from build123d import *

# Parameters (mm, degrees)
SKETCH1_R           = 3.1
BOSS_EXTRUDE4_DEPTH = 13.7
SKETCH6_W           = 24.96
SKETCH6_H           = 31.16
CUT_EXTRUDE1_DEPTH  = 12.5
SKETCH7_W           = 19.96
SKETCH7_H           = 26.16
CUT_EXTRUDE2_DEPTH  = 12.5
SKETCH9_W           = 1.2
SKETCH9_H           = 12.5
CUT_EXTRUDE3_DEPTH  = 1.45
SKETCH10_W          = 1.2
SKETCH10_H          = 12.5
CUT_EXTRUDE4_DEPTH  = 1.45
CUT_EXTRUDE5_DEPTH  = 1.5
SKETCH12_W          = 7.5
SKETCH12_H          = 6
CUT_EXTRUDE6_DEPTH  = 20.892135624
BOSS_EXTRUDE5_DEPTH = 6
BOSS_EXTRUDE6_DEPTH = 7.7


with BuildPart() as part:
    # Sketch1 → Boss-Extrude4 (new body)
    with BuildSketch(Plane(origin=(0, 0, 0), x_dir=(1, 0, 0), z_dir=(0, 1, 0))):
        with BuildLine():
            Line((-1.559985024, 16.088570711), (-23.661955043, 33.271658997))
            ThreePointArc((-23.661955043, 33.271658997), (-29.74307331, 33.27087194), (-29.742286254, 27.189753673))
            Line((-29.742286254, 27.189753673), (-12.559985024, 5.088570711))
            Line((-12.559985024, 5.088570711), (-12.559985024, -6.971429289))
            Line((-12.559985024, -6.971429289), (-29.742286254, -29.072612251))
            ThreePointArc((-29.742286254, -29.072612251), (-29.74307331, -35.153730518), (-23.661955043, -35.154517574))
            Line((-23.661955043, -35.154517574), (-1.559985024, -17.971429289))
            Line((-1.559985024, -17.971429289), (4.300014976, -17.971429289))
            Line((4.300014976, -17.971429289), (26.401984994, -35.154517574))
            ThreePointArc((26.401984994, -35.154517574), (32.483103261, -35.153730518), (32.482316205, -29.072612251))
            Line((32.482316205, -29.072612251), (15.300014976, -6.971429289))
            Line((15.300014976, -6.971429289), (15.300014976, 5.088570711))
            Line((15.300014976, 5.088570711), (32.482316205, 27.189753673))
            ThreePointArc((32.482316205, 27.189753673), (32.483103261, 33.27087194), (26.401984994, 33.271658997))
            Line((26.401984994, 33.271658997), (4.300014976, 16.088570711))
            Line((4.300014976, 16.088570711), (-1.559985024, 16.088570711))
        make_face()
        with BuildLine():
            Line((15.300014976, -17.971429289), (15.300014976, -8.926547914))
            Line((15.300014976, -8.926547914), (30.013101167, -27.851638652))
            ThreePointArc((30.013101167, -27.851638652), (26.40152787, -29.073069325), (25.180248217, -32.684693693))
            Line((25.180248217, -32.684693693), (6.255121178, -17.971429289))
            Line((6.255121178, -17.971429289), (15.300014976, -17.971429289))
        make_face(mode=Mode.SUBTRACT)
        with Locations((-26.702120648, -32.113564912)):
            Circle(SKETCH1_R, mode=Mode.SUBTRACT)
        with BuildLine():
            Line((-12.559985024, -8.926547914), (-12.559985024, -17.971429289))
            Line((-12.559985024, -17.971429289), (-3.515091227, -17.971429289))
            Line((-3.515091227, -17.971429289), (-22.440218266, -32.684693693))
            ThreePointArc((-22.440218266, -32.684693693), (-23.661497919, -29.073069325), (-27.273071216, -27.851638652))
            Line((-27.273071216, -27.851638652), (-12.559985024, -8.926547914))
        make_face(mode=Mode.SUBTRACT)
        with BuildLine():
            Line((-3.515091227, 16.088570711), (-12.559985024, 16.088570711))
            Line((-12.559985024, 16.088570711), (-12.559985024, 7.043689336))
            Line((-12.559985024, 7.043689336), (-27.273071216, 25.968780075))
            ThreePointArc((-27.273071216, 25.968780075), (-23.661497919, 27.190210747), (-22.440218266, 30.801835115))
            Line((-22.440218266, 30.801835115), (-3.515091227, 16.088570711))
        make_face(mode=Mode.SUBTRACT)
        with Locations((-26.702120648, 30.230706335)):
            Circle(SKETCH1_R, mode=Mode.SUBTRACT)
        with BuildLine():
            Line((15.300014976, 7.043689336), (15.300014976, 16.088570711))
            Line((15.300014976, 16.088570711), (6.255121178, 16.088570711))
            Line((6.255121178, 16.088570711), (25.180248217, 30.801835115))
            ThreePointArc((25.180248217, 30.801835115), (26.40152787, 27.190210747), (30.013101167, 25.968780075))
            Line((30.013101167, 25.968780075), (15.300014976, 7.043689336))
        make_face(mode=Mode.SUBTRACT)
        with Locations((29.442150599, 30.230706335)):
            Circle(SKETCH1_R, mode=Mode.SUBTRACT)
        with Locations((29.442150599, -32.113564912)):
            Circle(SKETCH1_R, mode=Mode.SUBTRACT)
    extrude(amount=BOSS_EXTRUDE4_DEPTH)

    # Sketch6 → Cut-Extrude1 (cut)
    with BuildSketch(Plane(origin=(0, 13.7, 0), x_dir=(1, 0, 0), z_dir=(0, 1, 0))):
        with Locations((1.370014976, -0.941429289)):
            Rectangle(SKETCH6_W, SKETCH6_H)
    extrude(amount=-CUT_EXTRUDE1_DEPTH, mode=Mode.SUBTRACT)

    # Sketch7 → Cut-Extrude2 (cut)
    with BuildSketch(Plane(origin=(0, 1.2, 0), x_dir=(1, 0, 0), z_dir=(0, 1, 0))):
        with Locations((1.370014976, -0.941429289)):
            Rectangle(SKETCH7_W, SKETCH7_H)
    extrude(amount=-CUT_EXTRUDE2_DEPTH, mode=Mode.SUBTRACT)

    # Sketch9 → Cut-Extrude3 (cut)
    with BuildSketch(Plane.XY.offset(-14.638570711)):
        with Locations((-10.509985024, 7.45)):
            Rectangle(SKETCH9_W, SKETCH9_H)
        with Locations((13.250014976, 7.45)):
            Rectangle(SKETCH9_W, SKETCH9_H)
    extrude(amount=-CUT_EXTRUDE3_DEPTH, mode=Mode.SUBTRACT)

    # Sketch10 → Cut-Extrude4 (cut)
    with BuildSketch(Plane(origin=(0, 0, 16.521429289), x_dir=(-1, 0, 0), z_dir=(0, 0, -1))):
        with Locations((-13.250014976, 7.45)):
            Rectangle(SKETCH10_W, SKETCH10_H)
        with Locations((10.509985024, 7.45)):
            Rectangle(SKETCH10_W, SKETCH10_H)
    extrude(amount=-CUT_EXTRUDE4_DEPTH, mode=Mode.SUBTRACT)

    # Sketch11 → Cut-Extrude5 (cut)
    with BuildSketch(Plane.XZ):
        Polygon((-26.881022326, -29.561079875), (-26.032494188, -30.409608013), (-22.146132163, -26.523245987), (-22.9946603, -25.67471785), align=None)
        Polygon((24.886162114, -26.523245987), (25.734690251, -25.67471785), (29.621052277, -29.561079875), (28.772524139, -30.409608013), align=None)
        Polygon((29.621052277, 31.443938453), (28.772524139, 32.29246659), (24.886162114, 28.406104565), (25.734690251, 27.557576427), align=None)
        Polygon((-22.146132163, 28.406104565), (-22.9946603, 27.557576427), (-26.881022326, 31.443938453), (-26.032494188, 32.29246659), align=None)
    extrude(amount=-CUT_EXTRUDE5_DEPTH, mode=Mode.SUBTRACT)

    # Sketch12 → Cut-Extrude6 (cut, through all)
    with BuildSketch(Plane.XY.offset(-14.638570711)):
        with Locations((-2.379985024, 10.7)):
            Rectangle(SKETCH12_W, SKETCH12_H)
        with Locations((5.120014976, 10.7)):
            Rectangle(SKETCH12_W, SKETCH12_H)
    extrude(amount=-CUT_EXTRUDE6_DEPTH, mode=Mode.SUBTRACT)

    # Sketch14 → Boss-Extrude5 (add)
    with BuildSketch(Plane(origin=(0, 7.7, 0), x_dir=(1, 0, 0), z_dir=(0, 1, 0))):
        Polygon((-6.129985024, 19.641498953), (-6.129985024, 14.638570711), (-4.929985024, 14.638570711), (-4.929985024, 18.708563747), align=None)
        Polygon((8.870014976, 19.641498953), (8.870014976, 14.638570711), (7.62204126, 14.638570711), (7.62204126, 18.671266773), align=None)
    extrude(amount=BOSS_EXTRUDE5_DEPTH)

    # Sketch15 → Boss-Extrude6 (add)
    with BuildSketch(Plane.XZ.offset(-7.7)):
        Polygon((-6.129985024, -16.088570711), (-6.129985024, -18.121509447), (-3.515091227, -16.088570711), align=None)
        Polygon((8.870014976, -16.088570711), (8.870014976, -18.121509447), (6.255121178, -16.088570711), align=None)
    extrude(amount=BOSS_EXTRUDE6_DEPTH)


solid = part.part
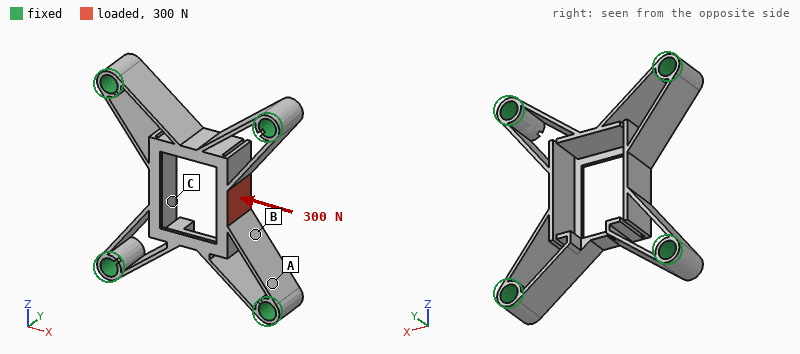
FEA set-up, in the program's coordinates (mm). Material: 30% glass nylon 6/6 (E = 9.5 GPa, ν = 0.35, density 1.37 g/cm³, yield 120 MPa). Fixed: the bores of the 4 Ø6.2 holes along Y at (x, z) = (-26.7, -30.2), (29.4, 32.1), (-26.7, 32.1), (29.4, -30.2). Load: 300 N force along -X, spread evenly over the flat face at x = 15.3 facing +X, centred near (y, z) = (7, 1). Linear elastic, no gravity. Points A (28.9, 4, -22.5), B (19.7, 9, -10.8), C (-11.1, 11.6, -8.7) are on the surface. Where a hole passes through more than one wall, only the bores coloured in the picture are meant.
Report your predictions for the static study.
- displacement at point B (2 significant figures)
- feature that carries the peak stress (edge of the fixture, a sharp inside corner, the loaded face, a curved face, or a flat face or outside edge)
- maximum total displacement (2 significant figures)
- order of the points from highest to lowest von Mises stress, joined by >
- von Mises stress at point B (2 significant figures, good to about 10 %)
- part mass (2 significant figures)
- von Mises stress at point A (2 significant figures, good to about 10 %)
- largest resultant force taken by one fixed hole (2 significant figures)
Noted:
0.037 mm
a flat face or outside edge
0.21 mm
B > A > C
23 MPa
10 g
11 MPa
240 N
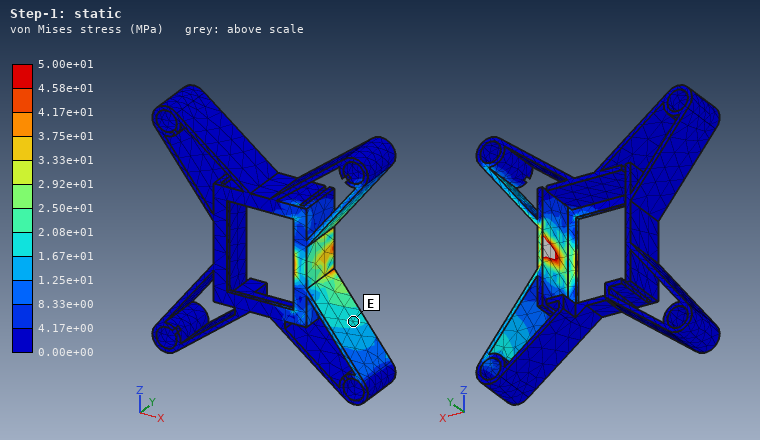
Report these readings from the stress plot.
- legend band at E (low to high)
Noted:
1.67e+01 to 2.08e+01 MPa
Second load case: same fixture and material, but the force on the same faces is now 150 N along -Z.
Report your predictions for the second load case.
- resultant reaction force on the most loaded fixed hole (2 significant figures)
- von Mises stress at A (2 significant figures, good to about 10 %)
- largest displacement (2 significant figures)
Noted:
77 N
3.9 MPa
0.19 mm
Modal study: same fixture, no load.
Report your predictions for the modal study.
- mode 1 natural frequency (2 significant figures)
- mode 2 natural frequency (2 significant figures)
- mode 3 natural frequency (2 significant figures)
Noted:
3100 Hz
3200 Hz
3600 Hz
